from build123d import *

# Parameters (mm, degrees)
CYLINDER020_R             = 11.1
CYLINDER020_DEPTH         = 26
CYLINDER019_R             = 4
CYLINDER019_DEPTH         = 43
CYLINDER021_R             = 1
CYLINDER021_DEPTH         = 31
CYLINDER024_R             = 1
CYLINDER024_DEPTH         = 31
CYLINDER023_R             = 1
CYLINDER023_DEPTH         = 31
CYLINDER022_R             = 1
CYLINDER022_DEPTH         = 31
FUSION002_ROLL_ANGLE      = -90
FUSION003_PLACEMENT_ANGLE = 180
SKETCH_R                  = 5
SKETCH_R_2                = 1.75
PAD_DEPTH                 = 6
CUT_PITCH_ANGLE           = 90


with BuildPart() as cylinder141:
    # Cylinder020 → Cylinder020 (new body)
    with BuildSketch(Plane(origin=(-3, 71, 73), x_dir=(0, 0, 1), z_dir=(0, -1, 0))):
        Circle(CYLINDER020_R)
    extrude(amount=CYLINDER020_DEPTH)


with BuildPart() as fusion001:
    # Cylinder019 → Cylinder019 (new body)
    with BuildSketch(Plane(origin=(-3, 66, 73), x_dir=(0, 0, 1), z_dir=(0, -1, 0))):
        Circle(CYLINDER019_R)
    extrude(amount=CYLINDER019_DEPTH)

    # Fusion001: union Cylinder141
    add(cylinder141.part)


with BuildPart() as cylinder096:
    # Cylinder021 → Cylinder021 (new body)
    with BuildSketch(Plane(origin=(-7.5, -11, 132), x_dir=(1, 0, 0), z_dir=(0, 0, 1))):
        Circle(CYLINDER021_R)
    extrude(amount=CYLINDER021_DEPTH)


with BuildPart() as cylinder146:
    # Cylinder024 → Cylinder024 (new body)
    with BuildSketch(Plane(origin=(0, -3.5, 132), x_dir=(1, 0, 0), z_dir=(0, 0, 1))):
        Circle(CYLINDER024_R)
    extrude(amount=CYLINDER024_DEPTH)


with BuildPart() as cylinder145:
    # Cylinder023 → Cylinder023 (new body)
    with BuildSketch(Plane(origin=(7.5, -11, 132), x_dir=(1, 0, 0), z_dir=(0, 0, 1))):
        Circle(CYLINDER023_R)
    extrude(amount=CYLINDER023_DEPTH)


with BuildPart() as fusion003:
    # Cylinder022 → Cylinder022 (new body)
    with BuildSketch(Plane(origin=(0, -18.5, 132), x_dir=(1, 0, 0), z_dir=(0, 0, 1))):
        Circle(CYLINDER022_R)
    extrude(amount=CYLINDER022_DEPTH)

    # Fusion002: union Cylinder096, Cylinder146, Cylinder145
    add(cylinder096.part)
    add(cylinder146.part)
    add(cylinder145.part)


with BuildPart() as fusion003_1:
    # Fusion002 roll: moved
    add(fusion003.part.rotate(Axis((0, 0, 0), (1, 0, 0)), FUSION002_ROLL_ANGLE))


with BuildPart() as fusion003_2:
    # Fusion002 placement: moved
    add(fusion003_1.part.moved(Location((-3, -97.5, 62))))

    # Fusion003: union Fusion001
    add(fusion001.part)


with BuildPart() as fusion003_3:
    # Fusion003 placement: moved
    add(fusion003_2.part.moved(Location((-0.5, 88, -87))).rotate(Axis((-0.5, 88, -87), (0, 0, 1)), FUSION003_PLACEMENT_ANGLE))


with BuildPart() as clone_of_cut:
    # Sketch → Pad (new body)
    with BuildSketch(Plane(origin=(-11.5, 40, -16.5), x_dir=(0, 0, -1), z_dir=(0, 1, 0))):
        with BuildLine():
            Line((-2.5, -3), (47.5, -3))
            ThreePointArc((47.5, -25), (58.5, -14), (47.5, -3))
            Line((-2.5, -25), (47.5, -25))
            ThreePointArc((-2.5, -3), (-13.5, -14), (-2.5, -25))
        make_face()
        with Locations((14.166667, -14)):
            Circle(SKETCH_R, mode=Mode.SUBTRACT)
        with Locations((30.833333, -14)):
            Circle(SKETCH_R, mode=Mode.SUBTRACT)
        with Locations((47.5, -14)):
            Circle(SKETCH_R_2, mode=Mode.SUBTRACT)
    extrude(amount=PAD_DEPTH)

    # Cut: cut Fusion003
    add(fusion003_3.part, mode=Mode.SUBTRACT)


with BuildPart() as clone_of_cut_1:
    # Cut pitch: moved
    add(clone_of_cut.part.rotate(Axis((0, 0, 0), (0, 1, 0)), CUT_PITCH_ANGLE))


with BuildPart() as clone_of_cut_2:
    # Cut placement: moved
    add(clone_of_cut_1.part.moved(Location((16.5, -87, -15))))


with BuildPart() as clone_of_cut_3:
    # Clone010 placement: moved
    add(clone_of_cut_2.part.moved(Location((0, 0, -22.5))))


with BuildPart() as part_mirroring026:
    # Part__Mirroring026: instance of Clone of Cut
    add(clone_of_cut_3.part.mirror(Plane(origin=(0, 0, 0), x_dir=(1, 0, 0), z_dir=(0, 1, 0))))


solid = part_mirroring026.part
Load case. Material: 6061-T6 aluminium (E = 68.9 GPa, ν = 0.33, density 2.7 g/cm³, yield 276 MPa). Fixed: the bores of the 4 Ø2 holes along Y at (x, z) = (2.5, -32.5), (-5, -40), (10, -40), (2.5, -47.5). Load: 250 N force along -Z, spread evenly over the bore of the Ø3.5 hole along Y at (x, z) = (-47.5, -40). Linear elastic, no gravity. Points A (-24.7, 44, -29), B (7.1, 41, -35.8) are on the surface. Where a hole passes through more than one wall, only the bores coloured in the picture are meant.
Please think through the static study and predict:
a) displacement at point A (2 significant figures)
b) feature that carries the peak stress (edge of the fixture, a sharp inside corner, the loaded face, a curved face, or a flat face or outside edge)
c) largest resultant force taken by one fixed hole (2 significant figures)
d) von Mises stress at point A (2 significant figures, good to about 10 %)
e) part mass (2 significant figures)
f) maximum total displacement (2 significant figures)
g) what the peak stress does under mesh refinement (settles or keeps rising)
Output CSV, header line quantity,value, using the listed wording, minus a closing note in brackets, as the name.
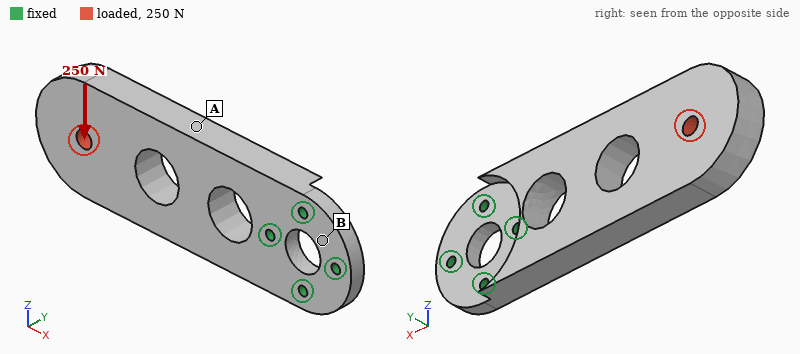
quantity,value
displacement at point A,25 µm
feature that carries the peak stress,edge of the fixture
largest resultant force taken by one fixed hole,560 N
von Mises stress at point A,16 MPa
part mass,18 g
maximum total displacement,67 µm
what the peak stress does under mesh refinement,keeps rising
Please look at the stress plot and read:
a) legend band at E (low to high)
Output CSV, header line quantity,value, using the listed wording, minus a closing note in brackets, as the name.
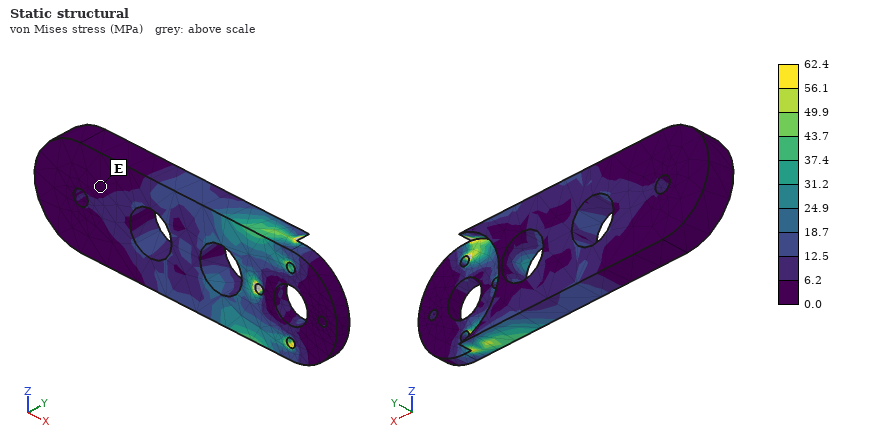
quantity,value
legend band at E,0.0 to 6.2 MPa
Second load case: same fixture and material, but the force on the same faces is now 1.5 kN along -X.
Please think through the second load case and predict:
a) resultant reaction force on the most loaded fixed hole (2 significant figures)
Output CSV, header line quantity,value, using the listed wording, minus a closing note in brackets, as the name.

quantity,value
resultant reaction force on the most loaded fixed hole,520 N
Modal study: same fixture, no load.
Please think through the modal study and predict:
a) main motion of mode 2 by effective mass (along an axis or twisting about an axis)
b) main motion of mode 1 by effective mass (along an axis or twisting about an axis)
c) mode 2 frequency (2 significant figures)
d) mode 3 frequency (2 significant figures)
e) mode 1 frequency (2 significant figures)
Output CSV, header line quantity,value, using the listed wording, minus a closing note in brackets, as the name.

quantity,value
main motion of mode 2 by effective mass,along Z
main motion of mode 1 by effective mass,along Y
mode 2 frequency,3800 Hz
mode 3 frequency,4800 Hz
mode 1 frequency,1100 Hz
